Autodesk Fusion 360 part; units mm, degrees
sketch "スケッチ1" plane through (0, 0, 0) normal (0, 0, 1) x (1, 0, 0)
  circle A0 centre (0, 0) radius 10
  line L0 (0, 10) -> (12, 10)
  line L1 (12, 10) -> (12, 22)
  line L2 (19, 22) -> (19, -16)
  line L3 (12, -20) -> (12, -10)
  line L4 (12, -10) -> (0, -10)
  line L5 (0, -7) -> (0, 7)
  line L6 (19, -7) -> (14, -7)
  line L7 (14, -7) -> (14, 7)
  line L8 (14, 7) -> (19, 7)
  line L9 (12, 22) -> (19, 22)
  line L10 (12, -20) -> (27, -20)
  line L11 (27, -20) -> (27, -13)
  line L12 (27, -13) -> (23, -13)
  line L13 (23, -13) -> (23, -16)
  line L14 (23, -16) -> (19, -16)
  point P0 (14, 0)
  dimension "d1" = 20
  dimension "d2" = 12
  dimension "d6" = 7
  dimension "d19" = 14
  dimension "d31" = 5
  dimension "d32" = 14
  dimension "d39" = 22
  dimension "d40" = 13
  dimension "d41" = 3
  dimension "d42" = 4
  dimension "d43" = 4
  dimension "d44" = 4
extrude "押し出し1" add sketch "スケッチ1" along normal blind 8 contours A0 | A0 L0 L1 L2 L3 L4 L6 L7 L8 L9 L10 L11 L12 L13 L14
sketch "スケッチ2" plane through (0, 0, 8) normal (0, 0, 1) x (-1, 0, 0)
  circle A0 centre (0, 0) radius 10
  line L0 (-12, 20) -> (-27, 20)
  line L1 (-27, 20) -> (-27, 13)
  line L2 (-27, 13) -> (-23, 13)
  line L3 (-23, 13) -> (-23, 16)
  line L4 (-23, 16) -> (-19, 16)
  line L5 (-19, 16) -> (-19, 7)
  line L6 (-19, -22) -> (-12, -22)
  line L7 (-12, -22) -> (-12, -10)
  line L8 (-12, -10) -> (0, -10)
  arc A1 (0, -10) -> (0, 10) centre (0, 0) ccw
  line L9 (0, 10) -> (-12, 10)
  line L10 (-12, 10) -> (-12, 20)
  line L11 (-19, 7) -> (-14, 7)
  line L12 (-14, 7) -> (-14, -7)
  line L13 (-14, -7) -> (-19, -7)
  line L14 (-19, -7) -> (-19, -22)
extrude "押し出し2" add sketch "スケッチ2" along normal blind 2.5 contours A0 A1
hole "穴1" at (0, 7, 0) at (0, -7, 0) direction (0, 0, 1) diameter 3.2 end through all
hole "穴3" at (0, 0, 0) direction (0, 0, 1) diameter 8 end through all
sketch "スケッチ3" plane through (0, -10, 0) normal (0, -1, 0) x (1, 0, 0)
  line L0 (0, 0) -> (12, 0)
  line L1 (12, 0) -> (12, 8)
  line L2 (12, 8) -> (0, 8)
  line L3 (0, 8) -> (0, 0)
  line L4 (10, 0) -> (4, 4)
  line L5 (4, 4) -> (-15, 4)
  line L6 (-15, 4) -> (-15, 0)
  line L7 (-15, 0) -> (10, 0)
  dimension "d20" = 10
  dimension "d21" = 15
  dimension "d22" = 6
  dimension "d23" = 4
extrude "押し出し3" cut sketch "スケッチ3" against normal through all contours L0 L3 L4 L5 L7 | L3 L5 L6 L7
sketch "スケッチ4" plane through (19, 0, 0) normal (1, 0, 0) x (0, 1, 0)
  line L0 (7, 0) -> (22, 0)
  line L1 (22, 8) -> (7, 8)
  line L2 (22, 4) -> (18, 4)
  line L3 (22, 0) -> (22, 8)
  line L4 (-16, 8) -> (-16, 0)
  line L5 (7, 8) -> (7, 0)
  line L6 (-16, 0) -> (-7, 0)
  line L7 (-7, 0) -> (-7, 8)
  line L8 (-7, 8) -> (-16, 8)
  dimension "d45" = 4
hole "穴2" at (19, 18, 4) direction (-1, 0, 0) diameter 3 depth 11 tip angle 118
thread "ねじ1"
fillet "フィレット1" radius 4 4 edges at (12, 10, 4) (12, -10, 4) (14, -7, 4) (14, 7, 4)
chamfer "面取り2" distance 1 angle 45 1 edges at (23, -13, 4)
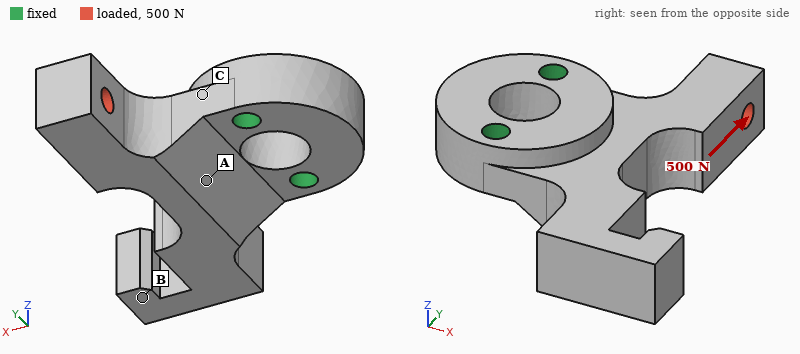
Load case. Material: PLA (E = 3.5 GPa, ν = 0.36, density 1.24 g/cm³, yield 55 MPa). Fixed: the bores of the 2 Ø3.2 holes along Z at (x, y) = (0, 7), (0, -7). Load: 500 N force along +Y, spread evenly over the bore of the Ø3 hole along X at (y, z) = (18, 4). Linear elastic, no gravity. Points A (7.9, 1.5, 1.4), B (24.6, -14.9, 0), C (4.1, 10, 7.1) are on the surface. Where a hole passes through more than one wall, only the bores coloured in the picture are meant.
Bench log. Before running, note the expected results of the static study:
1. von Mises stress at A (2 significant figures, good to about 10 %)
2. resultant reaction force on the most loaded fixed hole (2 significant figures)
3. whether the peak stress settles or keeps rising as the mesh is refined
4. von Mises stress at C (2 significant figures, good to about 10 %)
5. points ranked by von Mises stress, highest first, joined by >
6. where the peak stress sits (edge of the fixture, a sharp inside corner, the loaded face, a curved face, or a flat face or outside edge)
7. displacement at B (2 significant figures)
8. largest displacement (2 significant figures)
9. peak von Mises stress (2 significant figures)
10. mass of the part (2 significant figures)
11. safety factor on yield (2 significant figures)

11 MPa
570 N
settles
18 MPa
C > A > B
a curved face
0.12 mm
0.42 mm
47 MPa
5.6 g
1.2
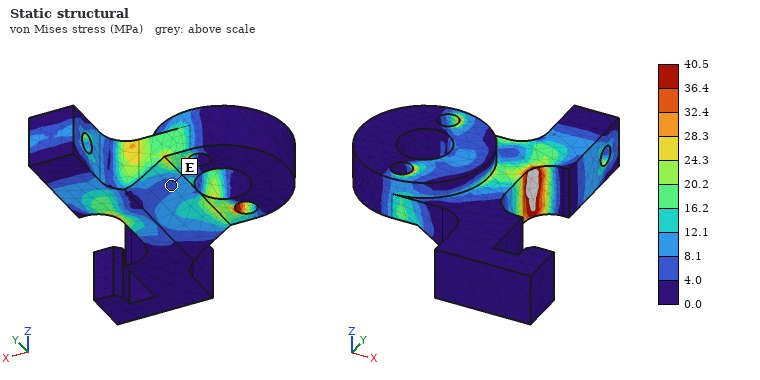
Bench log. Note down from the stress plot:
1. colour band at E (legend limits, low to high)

4.0 to 8.1 MPa
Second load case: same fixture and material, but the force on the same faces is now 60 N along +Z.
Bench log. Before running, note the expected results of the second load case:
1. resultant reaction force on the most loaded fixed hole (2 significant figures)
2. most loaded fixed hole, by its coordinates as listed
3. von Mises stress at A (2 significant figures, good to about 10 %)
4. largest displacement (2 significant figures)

93 N
(0, 7)
8.1 MPa
0.31 mm
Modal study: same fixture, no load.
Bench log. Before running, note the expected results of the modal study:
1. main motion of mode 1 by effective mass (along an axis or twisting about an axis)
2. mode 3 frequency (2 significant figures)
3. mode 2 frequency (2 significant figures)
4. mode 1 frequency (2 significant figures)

along Z
3300 Hz
2900 Hz
2000 Hz
